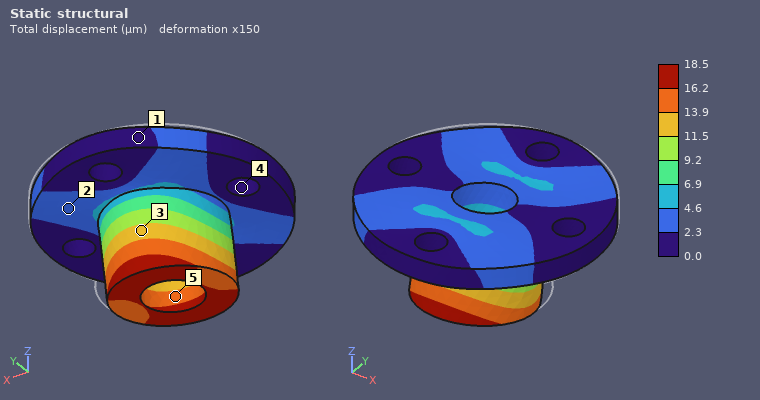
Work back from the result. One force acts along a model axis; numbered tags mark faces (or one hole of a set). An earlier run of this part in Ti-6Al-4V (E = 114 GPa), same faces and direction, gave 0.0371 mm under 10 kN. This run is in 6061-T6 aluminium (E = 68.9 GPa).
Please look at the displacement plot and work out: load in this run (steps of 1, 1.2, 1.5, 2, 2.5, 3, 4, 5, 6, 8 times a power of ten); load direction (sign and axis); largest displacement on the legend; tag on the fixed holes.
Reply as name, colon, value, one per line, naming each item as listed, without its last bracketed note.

load in this run: 3 kN
load direction: -Y
largest displacement on the legend: 18.5 µm
tag on the fixed holes: 4
